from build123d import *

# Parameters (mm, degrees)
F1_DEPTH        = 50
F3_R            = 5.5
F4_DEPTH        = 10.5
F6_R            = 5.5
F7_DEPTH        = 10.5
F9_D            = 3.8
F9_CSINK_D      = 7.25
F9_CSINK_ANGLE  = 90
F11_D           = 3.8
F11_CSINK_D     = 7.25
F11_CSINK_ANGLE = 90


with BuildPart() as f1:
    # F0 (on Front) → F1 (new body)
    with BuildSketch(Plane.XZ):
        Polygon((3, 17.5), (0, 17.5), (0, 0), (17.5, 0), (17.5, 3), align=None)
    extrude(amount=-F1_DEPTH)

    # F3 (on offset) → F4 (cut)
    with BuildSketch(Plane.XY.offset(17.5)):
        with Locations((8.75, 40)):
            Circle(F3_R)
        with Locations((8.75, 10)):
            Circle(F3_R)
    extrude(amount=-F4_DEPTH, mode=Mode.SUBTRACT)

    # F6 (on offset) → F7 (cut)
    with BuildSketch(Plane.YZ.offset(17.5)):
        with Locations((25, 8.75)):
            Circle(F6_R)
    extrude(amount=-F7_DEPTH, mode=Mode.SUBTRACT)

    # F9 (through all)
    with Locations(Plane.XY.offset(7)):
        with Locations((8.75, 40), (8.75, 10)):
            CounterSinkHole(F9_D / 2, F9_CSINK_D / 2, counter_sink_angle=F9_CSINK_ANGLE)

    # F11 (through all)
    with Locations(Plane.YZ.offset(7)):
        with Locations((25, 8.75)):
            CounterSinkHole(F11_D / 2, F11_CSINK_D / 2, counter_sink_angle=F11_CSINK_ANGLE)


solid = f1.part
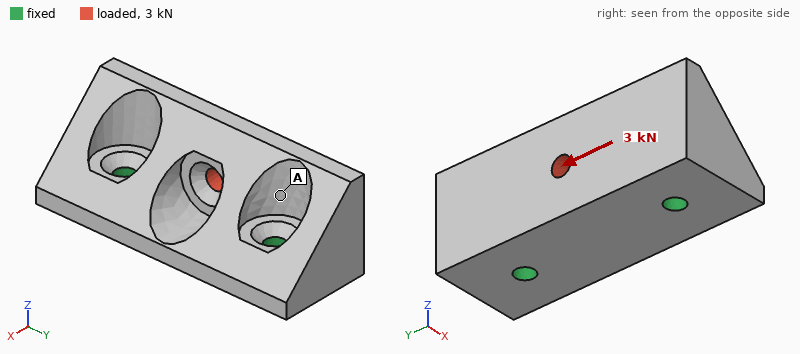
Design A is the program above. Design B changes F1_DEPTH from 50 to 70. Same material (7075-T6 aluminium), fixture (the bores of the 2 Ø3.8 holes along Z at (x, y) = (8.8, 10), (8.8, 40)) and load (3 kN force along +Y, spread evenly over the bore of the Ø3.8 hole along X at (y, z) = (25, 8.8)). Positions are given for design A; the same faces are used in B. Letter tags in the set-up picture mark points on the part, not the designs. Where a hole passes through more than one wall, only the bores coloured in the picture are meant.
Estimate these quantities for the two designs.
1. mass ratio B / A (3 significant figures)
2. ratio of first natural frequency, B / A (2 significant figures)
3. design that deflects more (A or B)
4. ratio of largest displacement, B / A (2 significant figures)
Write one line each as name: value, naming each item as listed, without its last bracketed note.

mass ratio B / A: 1.48
ratio of first natural frequency, B / A: 0.41
design that deflects more: B
ratio of largest displacement, B / A: 1.4
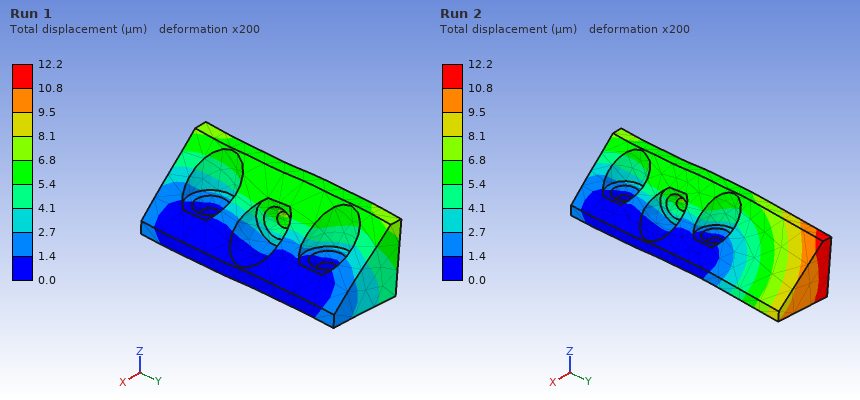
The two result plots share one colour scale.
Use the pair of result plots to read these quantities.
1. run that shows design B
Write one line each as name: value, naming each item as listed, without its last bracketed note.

run that shows design B: Run 2
